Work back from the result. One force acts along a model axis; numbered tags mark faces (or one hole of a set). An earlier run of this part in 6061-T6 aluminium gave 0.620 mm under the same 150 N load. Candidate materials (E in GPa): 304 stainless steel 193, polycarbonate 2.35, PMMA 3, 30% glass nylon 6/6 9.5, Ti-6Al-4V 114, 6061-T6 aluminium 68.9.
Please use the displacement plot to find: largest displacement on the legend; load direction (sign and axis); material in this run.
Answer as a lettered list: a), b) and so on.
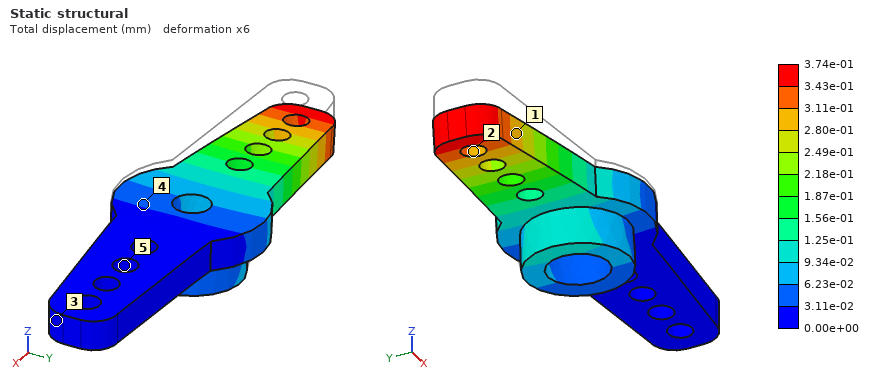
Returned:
a) 3.74e-01 mm
b) -Z
c) Ti-6Al-4V
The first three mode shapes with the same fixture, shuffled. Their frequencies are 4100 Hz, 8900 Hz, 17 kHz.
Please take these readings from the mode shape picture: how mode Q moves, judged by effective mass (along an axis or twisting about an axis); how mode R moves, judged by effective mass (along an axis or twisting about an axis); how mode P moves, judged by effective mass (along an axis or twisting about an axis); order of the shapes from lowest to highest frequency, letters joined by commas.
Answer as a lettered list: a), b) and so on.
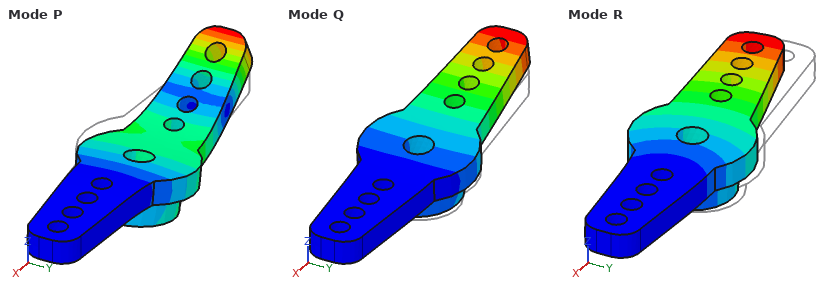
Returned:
a) along Z
b) along Y
c) along Z
d) Q, R, P
